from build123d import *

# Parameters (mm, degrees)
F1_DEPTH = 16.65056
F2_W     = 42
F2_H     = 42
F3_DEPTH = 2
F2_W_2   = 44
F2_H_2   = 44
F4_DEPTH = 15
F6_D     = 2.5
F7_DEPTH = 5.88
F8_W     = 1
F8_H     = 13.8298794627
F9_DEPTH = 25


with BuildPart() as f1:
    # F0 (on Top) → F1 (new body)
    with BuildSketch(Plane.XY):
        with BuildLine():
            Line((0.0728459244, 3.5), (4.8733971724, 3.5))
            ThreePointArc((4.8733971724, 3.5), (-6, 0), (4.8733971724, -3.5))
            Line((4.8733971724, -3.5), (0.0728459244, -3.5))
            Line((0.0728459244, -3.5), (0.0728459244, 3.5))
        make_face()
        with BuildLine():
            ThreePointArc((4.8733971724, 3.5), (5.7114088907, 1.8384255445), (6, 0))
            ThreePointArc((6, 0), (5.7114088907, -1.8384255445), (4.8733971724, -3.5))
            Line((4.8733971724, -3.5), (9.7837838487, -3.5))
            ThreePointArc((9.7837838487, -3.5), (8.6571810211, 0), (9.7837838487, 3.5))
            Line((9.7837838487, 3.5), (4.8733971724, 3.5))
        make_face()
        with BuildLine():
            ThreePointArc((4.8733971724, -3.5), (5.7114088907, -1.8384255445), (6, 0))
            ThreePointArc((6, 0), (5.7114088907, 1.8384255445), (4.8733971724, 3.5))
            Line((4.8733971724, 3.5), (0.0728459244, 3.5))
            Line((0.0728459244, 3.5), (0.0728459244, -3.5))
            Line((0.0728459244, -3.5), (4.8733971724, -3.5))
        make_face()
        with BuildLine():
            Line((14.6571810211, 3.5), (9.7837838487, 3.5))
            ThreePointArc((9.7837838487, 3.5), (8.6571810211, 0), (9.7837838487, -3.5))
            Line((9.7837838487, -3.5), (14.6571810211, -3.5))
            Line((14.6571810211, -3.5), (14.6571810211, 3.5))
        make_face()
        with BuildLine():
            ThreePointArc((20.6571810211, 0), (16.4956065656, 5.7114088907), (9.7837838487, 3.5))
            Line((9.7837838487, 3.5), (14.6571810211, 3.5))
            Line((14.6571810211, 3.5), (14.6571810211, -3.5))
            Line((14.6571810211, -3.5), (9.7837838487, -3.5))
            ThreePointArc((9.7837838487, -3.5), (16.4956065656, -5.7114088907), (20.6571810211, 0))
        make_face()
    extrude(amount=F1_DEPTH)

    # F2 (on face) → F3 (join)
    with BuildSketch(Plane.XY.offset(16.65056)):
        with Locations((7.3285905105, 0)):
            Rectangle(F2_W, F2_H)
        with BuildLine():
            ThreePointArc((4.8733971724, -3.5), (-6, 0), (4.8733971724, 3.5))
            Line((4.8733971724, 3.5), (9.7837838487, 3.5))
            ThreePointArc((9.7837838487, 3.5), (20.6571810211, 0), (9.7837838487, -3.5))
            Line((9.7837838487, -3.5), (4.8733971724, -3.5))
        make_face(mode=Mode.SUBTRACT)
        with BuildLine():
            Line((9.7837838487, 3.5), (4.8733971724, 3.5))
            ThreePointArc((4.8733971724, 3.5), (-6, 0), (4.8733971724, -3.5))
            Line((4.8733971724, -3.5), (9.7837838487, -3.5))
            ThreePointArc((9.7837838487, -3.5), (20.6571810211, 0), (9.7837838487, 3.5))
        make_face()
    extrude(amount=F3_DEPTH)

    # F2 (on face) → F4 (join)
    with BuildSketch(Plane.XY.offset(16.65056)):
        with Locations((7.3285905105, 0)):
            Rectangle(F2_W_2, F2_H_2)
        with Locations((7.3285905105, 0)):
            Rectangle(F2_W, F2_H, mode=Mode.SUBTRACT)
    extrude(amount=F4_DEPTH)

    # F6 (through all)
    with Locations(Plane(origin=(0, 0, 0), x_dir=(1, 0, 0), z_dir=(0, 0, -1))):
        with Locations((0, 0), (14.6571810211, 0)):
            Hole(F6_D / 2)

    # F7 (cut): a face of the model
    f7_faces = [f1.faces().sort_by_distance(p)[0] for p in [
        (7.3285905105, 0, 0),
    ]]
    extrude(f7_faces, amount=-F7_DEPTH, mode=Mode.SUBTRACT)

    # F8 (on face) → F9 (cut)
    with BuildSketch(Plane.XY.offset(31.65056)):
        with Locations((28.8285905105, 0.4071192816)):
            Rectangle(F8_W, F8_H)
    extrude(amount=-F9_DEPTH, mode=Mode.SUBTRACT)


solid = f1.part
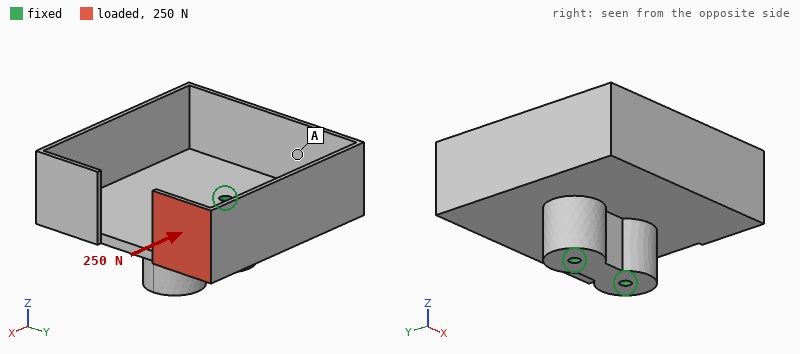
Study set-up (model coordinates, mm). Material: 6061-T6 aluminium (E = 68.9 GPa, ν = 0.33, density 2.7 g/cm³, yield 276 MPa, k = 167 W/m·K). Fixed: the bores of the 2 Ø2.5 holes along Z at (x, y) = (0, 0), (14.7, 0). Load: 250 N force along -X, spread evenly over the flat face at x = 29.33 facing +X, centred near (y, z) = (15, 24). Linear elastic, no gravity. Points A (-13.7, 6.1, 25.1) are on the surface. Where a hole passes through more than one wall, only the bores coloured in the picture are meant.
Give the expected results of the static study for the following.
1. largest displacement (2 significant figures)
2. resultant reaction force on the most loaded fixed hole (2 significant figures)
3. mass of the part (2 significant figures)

0.44 mm
280 N
23 g
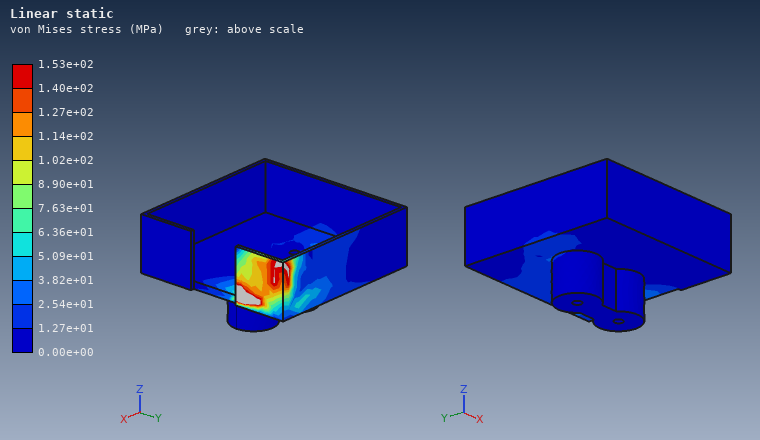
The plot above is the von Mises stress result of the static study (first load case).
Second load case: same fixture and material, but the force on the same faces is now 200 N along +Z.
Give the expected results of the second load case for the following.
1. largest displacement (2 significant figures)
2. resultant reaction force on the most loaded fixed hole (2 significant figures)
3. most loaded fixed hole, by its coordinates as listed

0.37 mm
270 N
(14.7, 0)
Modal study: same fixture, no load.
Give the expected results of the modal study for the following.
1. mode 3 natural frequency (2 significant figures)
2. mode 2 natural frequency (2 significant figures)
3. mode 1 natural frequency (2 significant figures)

2900 Hz
2800 Hz
2800 Hz
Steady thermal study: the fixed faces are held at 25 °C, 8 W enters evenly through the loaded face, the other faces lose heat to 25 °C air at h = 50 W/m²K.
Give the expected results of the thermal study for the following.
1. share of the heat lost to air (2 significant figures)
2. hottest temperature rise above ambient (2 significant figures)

18 %
30 K
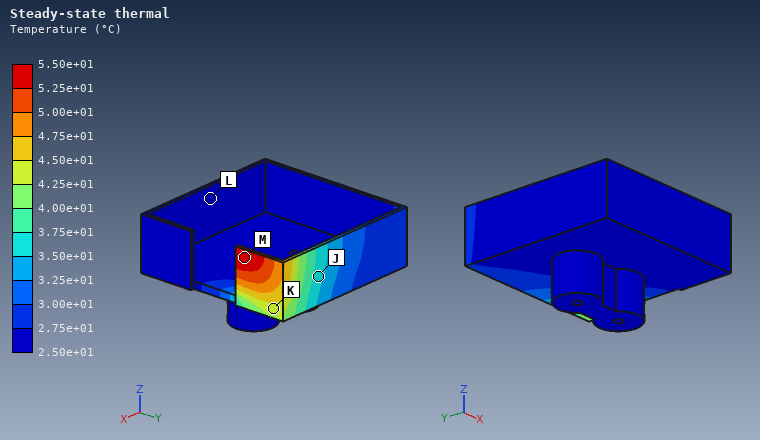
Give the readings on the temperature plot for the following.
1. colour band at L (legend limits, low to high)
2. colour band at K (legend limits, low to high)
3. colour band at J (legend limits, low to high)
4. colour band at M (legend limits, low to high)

2.50e+01 to 2.75e+01 °C
4.25e+01 to 4.50e+01 °C
3.50e+01 to 3.75e+01 °C
5.25e+01 to 5.50e+01 °C
